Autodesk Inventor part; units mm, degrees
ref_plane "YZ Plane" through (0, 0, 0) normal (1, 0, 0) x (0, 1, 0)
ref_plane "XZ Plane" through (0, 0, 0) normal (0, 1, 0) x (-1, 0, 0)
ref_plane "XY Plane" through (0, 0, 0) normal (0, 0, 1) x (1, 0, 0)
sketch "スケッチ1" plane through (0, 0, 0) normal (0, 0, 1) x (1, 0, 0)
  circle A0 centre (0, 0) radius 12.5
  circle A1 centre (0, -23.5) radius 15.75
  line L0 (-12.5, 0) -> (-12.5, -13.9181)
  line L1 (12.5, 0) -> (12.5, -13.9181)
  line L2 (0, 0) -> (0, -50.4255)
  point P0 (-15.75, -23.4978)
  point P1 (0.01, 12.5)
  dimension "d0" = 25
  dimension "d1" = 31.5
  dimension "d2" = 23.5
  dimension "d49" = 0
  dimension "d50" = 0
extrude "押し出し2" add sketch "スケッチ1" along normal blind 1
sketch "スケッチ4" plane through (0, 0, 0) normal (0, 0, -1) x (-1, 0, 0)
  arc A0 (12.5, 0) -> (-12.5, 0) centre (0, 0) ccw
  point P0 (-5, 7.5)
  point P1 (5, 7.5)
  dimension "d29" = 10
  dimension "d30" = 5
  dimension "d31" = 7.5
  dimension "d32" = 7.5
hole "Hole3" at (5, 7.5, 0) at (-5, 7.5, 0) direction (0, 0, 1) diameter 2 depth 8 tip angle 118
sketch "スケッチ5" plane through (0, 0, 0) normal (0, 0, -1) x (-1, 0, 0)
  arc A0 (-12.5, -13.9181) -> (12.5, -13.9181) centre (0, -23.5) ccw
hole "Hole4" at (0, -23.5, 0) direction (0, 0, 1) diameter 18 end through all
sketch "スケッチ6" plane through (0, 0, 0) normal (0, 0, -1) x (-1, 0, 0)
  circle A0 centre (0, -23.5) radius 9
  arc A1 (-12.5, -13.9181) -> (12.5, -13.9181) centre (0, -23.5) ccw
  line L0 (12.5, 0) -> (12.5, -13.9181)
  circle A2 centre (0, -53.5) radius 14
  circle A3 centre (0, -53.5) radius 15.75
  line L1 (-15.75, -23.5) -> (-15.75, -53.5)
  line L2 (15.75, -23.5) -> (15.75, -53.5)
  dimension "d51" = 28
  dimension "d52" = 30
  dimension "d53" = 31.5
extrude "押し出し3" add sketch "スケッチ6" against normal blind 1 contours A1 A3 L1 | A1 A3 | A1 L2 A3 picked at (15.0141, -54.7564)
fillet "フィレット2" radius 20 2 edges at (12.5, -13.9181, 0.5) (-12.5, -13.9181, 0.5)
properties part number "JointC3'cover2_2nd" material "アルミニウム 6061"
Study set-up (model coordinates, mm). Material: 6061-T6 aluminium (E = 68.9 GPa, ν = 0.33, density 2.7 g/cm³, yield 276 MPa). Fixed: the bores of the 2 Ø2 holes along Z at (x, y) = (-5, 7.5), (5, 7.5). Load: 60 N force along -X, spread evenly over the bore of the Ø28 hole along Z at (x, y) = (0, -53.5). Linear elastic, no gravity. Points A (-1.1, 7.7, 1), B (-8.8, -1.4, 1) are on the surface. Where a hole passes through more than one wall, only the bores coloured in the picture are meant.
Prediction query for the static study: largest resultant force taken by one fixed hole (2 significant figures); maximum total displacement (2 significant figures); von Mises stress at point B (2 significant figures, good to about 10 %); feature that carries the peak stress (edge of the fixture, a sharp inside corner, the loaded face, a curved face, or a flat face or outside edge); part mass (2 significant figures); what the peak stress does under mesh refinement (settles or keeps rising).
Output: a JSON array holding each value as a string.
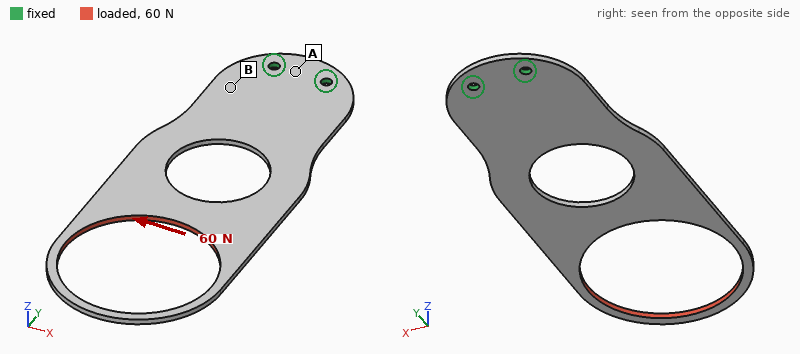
["320 N", "0.33 mm", "23 MPa", "edge of the fixture", "3.6 g", "keeps rising"]
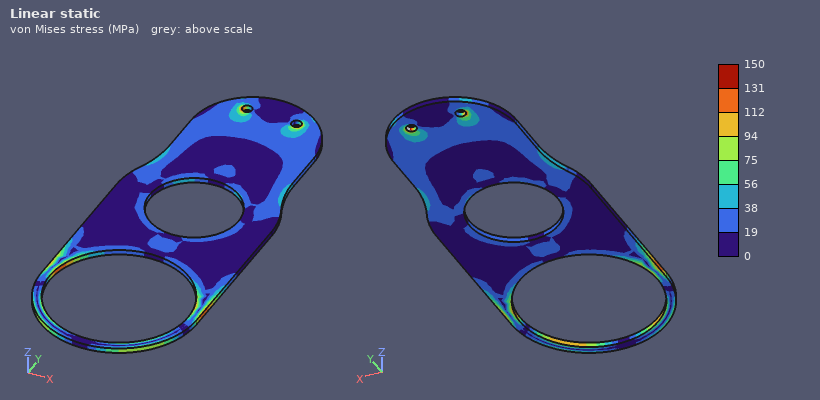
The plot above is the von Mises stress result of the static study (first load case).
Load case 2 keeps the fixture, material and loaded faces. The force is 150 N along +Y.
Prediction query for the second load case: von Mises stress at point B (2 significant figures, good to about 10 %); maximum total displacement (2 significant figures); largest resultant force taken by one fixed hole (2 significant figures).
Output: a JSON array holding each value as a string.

["7.1 MPa", "81 µm", "75 N"]
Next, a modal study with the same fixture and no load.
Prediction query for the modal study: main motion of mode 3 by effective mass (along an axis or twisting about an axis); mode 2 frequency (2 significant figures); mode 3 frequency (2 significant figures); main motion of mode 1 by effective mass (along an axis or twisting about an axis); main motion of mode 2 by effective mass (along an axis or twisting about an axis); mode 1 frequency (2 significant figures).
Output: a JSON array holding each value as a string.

["along Z", "730 Hz", "880 Hz", "along Z", "twisting about Y", "220 Hz"]
